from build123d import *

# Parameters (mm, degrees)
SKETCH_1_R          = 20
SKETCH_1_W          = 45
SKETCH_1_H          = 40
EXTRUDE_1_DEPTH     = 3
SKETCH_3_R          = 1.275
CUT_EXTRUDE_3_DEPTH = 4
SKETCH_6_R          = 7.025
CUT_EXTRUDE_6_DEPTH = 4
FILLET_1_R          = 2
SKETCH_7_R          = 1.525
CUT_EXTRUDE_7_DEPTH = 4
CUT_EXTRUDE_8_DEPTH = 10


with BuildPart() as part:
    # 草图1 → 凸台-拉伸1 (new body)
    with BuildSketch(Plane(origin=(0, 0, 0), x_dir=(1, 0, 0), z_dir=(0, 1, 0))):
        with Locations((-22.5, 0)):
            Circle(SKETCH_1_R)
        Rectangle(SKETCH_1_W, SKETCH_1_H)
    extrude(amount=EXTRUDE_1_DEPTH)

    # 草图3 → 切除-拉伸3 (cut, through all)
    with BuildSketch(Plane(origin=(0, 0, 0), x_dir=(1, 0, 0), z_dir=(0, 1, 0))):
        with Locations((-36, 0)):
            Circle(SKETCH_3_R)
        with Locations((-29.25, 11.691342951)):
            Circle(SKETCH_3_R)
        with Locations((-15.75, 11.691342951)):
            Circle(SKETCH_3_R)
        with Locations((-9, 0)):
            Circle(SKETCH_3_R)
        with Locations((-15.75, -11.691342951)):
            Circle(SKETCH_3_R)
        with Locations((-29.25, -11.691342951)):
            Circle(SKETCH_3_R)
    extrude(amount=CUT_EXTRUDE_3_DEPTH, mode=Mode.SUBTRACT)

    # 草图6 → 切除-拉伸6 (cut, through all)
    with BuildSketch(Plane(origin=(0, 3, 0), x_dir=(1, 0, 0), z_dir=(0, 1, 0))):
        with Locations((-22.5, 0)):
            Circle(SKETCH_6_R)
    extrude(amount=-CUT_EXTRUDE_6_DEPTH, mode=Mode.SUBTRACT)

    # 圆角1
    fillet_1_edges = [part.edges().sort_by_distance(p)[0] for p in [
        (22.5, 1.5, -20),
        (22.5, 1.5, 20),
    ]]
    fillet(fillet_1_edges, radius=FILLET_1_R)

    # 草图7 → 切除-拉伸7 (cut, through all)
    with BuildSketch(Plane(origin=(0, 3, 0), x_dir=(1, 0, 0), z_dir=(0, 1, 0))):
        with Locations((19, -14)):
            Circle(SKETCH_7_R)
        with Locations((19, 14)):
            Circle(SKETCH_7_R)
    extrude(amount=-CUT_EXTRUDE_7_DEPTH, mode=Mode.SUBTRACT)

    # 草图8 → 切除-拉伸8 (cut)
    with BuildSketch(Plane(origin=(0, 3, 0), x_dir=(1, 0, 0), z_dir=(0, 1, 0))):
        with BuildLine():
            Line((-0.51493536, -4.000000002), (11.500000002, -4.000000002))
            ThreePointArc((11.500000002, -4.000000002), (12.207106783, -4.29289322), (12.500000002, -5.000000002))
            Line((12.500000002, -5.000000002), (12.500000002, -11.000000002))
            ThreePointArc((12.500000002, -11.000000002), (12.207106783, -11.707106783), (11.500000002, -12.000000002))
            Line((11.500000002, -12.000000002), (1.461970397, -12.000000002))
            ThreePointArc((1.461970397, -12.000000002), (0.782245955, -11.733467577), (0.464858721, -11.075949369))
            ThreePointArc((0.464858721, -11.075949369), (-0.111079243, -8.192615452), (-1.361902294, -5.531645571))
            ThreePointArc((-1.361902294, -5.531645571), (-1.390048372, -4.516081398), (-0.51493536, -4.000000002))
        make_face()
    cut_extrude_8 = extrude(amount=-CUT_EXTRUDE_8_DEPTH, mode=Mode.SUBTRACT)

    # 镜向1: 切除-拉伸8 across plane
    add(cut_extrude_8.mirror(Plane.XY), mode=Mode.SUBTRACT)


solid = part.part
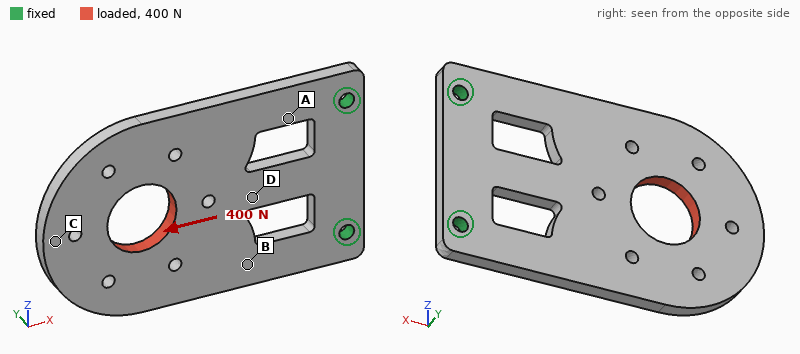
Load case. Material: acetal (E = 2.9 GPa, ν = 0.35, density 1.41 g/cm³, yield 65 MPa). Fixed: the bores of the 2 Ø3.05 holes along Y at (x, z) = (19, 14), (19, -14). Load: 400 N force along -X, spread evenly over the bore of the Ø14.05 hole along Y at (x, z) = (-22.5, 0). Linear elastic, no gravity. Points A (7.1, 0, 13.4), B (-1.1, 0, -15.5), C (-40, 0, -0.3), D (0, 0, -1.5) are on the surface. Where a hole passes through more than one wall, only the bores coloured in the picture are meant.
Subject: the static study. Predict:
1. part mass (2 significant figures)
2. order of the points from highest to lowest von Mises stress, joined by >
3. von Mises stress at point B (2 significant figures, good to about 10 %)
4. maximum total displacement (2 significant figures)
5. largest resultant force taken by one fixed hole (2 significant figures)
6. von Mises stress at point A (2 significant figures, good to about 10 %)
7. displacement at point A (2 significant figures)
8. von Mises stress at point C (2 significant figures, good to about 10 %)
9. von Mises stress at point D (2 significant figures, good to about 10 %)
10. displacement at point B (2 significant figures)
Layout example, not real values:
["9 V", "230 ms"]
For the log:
["8.6 g", "A > B > D > C", "5.5 MPa", "0.11 mm", "200 N", "7.2 MPa", "0.029 mm", "2.3 MPa", "4.0 MPa", "0.047 mm"]
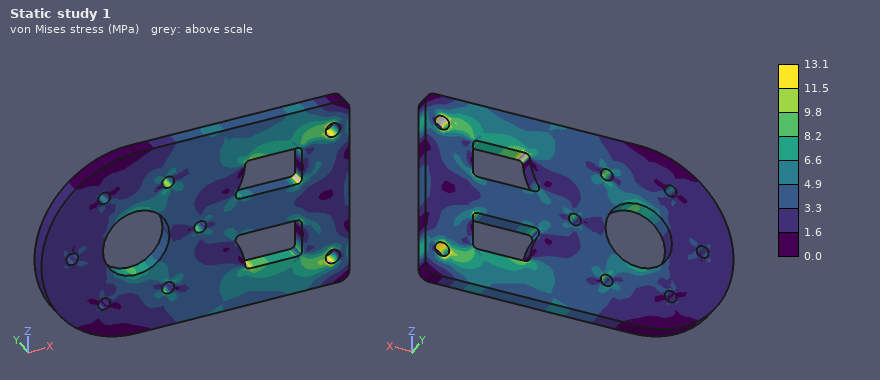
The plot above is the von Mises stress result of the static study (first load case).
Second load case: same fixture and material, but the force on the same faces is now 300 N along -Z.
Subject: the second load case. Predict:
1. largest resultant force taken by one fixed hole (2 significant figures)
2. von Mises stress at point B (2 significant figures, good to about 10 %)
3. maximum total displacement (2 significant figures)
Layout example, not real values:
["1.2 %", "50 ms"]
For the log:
["430 N", "8.1 MPa", "0.75 mm"]
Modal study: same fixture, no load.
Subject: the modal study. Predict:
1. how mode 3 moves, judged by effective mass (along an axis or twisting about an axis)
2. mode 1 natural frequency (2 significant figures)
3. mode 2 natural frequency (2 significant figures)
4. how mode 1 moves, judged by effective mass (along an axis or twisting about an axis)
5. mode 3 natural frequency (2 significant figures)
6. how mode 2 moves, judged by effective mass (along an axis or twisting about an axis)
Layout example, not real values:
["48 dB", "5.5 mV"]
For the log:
["along Y", "180 Hz", "650 Hz", "along Y", "1100 Hz", "twisting about X"]
